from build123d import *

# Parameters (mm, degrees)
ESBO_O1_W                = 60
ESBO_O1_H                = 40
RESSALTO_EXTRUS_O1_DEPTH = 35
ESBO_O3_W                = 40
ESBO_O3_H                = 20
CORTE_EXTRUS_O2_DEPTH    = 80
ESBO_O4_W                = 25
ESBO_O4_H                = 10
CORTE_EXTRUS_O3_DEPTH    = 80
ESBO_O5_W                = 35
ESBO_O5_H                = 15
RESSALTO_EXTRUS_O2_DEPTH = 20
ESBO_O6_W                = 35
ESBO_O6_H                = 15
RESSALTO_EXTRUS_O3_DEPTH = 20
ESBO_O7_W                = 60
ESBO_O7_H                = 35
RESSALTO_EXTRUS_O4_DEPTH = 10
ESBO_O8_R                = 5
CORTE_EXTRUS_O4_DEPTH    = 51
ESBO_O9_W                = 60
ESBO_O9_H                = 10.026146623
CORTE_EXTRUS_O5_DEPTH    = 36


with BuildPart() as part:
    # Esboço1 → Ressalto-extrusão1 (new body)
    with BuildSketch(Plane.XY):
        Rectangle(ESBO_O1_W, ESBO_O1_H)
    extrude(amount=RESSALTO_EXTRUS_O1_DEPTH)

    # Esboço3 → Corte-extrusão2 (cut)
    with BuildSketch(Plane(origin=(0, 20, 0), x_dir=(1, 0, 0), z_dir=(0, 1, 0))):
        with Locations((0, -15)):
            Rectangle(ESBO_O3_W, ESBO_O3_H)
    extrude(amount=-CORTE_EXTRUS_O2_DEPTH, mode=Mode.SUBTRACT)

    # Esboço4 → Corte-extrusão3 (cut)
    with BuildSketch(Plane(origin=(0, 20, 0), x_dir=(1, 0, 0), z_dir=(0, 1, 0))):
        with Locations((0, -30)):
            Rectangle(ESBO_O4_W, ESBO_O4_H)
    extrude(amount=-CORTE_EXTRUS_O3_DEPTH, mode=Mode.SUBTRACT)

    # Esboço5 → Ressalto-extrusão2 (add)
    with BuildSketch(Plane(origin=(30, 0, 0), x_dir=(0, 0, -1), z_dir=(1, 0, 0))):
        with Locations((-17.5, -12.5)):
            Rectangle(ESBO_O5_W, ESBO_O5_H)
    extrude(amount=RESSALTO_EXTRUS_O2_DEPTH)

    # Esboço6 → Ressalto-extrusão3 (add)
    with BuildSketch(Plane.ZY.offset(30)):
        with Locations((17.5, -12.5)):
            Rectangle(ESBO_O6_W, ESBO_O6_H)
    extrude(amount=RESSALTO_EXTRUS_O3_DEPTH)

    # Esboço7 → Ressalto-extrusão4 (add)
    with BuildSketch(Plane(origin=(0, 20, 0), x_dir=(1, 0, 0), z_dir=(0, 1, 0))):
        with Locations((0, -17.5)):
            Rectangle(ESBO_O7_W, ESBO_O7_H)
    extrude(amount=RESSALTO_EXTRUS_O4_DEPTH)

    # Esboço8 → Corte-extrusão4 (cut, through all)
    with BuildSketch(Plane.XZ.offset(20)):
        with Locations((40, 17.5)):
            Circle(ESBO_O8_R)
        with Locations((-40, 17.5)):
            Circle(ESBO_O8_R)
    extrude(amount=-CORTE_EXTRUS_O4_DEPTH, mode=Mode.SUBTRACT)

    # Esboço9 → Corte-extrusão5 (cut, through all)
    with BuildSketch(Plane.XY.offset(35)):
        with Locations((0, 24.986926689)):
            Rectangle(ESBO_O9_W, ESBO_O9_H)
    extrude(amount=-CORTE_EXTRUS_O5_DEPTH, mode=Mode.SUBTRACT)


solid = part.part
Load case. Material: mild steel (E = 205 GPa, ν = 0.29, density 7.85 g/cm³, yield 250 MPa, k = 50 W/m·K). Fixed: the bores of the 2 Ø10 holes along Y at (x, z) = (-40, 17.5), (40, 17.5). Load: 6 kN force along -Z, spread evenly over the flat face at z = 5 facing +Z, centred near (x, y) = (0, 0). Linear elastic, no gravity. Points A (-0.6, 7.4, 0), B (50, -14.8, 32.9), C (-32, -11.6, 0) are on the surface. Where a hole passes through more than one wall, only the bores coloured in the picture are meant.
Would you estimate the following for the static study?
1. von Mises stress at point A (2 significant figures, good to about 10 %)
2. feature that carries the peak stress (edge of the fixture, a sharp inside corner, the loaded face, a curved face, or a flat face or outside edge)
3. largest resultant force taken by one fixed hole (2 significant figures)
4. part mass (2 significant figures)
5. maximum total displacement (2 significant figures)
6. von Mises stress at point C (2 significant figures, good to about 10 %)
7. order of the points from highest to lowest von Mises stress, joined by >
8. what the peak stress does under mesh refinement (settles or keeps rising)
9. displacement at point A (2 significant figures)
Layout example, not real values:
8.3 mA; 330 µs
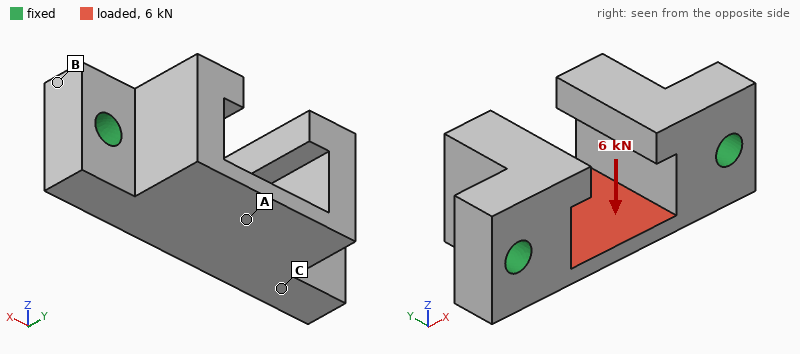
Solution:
80 MPa; edge of the fixture; 3.7 kN; 480 g; 38 µm; 24 MPa; A > C > B; keeps rising; 31 µm
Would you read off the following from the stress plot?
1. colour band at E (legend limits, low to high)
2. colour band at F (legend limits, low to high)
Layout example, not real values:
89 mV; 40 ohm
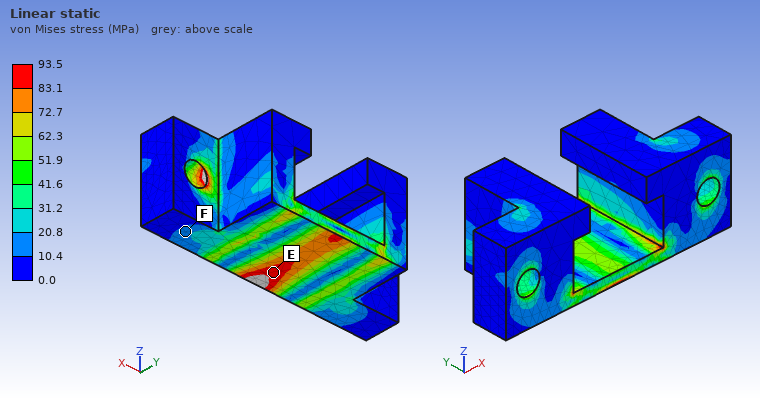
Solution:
83.1 to 93.5 MPa; 10.4 to 20.8 MPa
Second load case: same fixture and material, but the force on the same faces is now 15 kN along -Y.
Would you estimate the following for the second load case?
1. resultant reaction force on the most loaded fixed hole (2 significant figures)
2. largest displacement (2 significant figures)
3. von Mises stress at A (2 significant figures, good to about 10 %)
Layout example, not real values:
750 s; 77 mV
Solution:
7.8 kN; 31 µm; 46 MPa
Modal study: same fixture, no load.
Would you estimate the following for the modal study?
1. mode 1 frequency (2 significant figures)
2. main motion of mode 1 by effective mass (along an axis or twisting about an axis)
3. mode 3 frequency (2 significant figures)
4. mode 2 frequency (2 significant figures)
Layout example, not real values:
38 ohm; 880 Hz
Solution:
6900 Hz; along Z; 8100 Hz; 7400 Hz
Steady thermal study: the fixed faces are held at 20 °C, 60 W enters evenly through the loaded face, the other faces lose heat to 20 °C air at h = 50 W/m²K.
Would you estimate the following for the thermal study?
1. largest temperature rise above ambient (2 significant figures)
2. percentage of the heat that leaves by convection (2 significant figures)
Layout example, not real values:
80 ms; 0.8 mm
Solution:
64 K; 22 %
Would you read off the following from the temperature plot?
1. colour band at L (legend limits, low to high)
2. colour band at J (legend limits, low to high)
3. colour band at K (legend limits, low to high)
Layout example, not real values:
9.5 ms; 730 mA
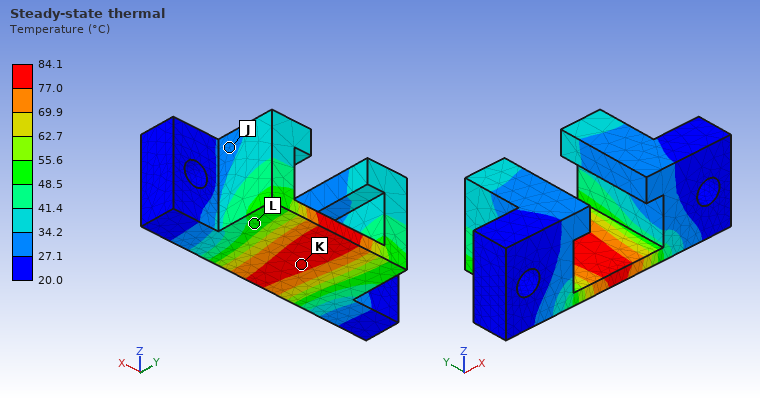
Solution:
48.5 to 55.6 °C; 27.1 to 34.2 °C; 77.0 to 84.1 °C
